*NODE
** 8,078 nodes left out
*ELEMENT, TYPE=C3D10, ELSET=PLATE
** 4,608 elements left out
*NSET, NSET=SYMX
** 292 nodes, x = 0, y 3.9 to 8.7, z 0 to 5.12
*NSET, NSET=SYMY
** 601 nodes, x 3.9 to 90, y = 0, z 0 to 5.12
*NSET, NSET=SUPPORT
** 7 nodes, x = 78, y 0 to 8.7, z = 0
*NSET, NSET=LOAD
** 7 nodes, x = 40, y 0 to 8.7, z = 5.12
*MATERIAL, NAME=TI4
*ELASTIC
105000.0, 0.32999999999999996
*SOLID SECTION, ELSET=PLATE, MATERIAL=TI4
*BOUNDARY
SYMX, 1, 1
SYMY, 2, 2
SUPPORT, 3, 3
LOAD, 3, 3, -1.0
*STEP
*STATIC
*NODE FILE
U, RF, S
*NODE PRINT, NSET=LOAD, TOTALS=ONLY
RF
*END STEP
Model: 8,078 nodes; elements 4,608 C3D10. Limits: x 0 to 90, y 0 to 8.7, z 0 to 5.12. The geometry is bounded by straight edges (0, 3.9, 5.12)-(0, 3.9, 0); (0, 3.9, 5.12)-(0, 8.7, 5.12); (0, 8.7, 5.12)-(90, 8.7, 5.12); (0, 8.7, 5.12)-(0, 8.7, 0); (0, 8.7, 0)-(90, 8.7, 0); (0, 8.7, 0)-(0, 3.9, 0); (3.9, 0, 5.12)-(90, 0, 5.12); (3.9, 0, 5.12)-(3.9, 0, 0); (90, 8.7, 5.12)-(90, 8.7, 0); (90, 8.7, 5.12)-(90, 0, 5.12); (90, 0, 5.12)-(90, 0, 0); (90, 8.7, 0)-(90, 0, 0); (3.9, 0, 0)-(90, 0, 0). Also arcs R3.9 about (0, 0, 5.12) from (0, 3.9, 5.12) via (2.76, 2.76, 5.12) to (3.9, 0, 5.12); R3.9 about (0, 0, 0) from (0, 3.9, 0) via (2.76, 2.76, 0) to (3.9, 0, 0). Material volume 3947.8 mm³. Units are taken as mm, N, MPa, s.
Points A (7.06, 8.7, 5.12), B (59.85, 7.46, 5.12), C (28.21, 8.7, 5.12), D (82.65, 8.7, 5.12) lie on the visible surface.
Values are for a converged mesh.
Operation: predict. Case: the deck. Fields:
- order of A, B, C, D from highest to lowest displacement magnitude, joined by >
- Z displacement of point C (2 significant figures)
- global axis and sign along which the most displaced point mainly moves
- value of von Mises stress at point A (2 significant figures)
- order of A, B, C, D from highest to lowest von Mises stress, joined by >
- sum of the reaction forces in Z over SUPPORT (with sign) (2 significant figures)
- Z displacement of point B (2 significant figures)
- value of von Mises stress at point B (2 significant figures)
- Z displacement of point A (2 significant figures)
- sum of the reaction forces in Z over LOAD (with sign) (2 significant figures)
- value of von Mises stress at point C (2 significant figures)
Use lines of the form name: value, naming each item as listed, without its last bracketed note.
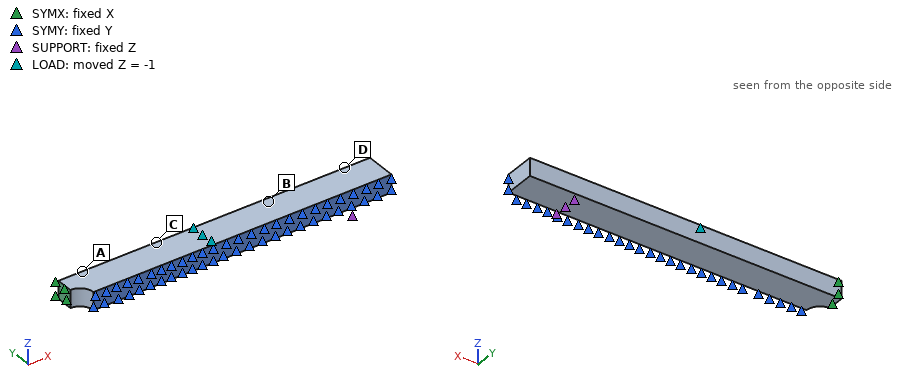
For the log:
order of A, B, C, D from highest to lowest displacement magnitude, joined by >: A > C > B > D
Z displacement of point C: -1.2 mm
global axis and sign along which the most displaced point mainly moves: -Z
value of von Mises stress at point A: 150 MPa
order of A, B, C, D from highest to lowest von Mises stress, joined by >: A > C > B > D
sum of the reaction forces in Z over SUPPORT (with sign): 130 N
Z displacement of point B: -0.52 mm
value of von Mises stress at point B: 60 MPa
Z displacement of point A: -1.4 mm
sum of the reaction forces in Z over LOAD (with sign): -130 N
value of von Mises stress at point C: 130 MPa
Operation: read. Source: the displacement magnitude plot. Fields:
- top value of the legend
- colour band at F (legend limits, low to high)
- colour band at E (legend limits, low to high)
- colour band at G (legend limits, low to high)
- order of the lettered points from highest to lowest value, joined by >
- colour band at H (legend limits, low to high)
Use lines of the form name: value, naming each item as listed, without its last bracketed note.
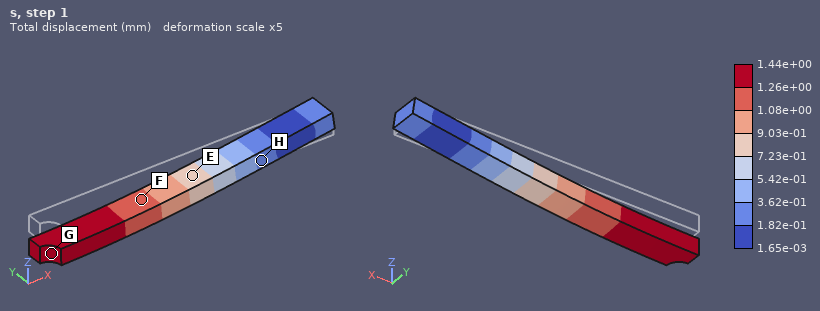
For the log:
top value of the legend: 1.44e+00 mm
colour band at F: 1.08e+00 to 1.26e+00 mm
colour band at E: 7.23e-01 to 9.03e-01 mm
colour band at G: 1.26e+00 to 1.44e+00 mm
order of the lettered points from highest to lowest value, joined by >: G > F > E > H
colour band at H: 1.82e-01 to 3.62e-01 mm
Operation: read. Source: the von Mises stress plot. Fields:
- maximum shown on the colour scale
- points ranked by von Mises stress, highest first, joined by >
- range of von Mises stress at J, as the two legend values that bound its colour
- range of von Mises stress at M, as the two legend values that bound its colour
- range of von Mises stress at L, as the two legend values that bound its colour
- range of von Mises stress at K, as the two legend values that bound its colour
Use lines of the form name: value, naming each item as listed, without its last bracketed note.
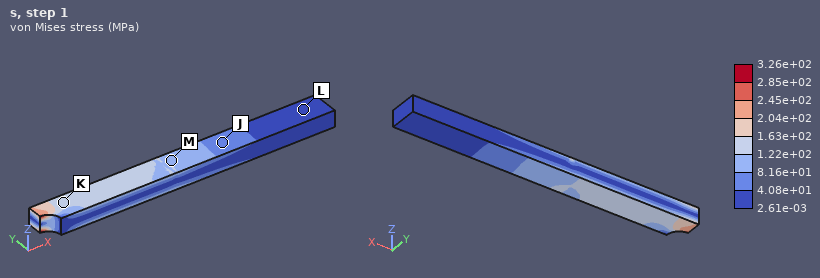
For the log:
maximum shown on the colour scale: 3.26e+02 MPa
points ranked by von Mises stress, highest first, joined by >: K > M > J > L
range of von Mises stress at J, as the two legend values that bound its colour: 4.08e+01 to 8.16e+01 MPa
range of von Mises stress at M, as the two legend values that bound its colour: 8.16e+01 to 1.22e+02 MPa
range of von Mises stress at L, as the two legend values that bound its colour: 2.61e-03 to 4.08e+01 MPa
range of von Mises stress at K, as the two legend values that bound its colour: 1.22e+02 to 1.63e+02 MPa
